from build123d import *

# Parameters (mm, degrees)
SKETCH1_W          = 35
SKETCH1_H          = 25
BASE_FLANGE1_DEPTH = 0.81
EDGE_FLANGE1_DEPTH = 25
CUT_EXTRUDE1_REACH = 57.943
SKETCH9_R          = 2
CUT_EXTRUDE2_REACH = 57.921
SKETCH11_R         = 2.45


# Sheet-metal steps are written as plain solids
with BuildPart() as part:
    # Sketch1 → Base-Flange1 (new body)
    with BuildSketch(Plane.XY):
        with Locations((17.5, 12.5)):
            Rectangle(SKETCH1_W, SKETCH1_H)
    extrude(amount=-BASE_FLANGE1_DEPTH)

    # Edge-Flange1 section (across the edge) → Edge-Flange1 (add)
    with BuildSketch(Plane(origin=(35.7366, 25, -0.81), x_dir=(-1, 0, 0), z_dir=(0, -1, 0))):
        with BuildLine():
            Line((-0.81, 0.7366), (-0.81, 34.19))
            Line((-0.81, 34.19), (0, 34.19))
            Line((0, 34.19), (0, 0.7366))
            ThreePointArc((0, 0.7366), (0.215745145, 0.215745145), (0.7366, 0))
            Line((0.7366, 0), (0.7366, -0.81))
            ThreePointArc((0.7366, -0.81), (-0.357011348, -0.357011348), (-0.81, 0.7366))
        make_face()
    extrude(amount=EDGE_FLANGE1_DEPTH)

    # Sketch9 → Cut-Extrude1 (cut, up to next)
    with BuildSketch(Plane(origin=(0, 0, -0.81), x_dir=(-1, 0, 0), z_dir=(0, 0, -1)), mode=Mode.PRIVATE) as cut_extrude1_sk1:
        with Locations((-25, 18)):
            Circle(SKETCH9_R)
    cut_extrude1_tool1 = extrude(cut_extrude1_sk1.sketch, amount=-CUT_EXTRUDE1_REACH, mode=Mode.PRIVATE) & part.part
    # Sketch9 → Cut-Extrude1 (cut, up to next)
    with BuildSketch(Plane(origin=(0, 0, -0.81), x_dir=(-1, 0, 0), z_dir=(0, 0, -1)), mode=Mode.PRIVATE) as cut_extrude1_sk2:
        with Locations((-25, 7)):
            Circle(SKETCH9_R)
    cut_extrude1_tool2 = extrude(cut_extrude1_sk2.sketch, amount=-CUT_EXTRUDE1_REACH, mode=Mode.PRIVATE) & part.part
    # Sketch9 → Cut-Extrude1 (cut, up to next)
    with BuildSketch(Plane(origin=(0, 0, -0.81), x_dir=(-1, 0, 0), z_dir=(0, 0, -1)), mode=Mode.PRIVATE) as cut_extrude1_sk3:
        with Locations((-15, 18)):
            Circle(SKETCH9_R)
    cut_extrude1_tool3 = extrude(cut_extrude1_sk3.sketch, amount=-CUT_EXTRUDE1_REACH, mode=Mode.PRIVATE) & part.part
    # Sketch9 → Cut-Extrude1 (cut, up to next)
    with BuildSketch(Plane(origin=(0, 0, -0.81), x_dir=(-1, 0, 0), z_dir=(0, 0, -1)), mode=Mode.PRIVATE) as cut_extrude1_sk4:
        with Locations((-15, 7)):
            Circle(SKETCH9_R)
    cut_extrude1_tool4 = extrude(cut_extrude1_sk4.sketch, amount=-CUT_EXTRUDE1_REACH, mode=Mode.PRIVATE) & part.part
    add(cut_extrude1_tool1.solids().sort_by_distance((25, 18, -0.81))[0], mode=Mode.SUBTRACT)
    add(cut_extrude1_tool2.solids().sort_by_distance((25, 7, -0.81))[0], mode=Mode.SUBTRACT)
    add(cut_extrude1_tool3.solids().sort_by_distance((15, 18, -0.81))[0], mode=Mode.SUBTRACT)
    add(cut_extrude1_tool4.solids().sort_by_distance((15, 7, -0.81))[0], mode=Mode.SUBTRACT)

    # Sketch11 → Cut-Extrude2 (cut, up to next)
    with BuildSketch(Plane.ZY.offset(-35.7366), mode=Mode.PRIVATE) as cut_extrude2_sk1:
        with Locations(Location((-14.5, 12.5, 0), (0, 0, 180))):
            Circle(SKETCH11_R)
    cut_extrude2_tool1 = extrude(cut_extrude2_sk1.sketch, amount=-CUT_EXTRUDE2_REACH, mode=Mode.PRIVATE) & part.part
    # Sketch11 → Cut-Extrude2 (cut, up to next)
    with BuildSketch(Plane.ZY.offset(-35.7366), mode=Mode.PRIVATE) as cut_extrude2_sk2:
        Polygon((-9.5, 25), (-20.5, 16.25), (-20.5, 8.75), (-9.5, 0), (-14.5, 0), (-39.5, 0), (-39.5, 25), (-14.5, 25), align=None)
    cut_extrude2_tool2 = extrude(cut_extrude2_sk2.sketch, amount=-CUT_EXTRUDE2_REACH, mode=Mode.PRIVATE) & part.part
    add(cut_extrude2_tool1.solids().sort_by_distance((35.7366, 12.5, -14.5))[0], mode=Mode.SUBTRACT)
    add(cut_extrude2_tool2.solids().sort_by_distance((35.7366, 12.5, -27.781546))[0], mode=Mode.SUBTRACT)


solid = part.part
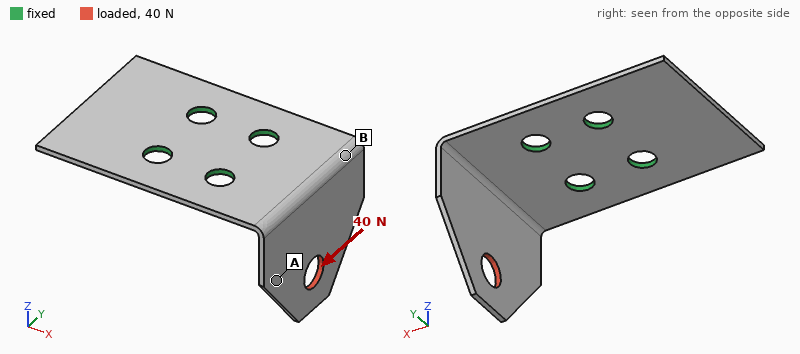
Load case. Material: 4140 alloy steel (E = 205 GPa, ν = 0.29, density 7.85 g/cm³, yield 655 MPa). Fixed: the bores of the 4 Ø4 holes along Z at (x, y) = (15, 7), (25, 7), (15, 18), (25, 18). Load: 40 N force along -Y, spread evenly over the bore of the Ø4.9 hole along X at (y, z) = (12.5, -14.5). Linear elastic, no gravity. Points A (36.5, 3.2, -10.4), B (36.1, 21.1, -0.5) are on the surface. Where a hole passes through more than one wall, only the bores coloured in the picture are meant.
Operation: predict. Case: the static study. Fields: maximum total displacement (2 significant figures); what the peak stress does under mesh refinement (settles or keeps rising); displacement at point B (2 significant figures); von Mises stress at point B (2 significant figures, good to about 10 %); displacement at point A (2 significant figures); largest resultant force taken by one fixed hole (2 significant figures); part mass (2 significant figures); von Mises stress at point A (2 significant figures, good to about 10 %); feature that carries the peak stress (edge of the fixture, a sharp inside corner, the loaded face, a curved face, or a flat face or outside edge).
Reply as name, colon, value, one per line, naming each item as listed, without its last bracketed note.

maximum total displacement: 0.13 mm
what the peak stress does under mesh refinement: keeps rising
displacement at point B: 0.052 mm
von Mises stress at point B: 66 MPa
displacement at point A: 0.087 mm
largest resultant force taken by one fixed hole: 49 N
part mass: 7.8 g
von Mises stress at point A: 19 MPa
feature that carries the peak stress: edge of the fixture
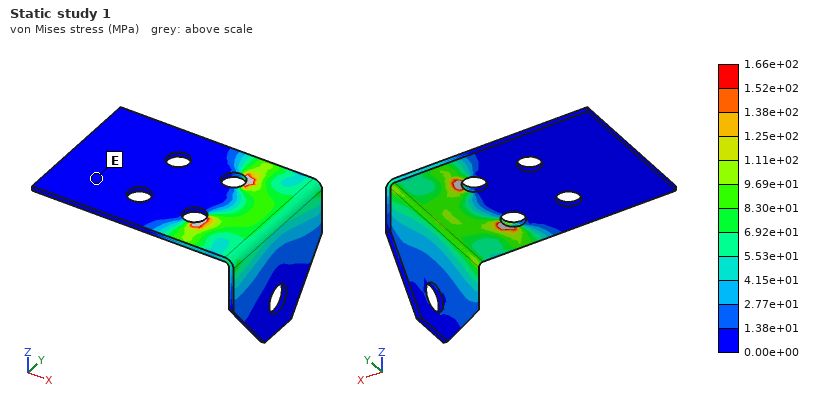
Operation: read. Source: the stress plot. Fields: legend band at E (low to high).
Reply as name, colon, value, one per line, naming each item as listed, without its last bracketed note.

legend band at E: 0.00e+00 to 1.38e+01 MPa
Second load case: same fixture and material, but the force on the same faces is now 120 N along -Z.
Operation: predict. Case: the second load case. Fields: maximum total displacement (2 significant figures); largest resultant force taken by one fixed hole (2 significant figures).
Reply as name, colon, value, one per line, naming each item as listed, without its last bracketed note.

maximum total displacement: 0.52 mm
largest resultant force taken by one fixed hole: 64 N
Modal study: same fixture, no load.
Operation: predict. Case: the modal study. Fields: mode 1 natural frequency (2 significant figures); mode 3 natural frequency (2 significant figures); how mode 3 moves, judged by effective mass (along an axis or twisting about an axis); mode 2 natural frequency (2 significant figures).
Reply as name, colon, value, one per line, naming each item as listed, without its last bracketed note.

mode 1 natural frequency: 1300 Hz
mode 3 natural frequency: 3600 Hz
how mode 3 moves, judged by effective mass: along Z
mode 2 natural frequency: 2500 Hz
